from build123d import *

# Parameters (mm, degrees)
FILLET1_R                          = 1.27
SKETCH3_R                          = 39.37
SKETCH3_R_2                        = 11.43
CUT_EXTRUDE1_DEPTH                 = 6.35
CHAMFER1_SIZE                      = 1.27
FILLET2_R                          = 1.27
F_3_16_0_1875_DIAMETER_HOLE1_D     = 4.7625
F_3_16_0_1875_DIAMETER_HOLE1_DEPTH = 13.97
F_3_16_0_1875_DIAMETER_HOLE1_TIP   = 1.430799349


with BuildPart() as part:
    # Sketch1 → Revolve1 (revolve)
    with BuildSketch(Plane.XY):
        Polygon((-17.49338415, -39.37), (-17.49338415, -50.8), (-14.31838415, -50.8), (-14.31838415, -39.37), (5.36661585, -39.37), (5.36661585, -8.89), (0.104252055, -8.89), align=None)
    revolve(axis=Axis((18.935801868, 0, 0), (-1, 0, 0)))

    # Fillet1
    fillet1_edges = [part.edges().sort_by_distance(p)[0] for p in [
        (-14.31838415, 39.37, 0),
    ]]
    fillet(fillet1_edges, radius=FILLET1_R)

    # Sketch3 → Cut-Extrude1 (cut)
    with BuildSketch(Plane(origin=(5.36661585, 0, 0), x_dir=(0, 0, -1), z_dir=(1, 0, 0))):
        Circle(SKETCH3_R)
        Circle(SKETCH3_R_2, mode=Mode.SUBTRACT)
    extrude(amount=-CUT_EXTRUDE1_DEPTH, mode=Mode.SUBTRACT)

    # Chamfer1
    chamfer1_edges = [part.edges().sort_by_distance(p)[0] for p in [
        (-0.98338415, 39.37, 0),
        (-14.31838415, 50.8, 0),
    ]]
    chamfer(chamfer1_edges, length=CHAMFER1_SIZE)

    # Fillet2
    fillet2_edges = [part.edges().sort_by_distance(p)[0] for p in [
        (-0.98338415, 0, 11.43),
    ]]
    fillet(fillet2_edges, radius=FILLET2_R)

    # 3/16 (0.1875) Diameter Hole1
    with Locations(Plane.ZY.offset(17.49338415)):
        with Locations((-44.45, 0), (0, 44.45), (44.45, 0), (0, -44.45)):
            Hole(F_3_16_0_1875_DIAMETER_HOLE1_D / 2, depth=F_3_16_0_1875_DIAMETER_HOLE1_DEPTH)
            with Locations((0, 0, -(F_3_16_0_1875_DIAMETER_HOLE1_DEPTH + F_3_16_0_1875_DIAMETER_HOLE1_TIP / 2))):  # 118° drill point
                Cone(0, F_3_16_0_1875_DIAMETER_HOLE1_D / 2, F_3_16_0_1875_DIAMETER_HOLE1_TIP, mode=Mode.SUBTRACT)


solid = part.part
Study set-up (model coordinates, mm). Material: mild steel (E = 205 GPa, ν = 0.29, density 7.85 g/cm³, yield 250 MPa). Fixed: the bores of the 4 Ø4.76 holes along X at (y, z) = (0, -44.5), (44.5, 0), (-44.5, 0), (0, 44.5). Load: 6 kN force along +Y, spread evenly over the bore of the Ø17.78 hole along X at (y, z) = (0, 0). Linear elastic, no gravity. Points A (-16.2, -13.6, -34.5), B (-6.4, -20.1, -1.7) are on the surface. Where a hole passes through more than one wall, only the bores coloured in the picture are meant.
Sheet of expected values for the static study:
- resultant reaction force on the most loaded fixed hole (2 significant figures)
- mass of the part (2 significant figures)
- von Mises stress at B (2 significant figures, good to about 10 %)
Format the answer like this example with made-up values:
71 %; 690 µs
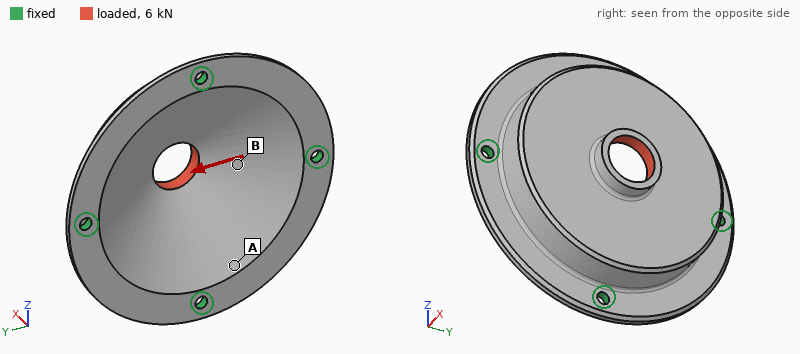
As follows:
2.4 kN; 430 g; 39 MPa
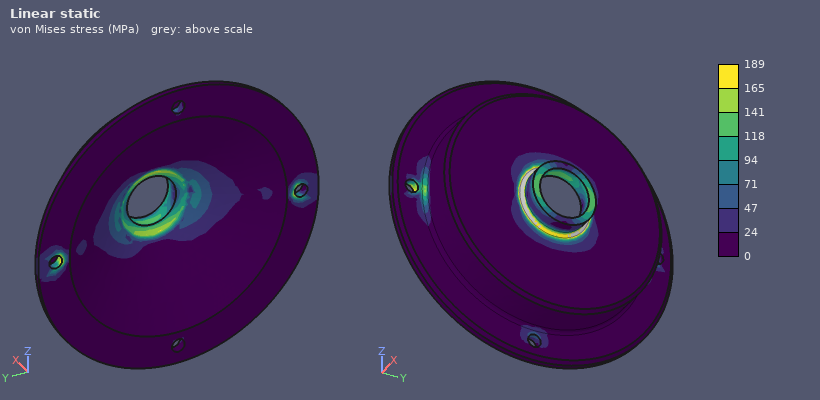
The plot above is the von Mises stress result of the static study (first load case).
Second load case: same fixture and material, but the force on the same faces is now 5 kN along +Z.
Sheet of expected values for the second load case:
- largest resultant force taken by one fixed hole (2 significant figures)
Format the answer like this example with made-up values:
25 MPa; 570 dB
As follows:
2.0 kN
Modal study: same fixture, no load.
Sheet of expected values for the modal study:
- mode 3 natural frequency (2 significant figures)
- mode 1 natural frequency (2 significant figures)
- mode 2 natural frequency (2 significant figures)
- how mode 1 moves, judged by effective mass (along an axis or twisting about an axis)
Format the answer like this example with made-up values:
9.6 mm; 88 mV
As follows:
7700 Hz; 7300 Hz; 7700 Hz; along X
